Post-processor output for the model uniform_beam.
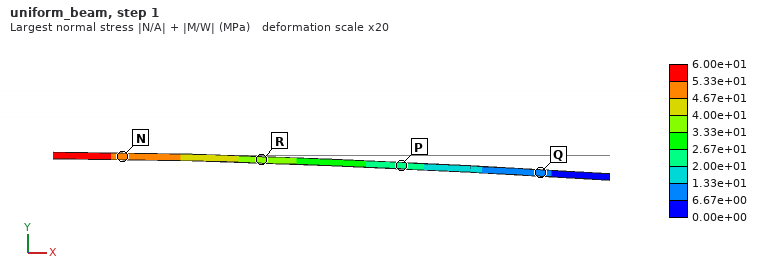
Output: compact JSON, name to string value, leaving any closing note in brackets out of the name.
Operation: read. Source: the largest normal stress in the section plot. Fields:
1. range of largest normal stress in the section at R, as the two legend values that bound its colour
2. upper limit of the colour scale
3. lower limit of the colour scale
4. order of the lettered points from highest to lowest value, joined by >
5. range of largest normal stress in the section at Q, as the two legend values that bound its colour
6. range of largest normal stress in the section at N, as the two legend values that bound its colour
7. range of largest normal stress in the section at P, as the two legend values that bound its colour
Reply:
{"range of largest normal stress in the section at R, as the two legend values that bound its colour": "3.33e+01 to 4.00e+01 MPa", "upper limit of the colour scale": "6.00e+01 MPa", "lower limit of the colour scale": "0.00e+00 MPa", "order of the lettered points from highest to lowest value, joined by >": "N > R > P > Q", "range of largest normal stress in the section at Q, as the two legend values that bound its colour": "6.67e+00 to 1.33e+01 MPa", "range of largest normal stress in the section at N, as the two legend values that bound its colour": "4.67e+01 to 5.33e+01 MPa", "range of largest normal stress in the section at P, as the two legend values that bound its colour": "2.00e+01 to 2.67e+01 MPa"}
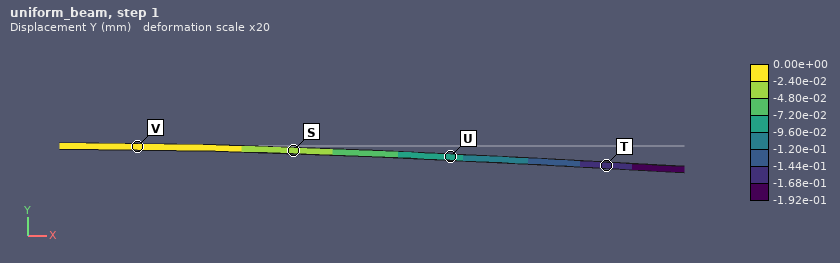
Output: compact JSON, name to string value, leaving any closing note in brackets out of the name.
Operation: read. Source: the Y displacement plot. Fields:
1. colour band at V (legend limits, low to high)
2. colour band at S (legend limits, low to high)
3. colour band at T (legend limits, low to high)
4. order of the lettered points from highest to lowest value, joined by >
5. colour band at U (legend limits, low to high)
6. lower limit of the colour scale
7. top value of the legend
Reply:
{"colour band at V": "-2.40e-02 to 0.00e+00 mm", "colour band at S": "-4.80e-02 to -2.40e-02 mm", "colour band at T": "-1.68e-01 to -1.44e-01 mm", "order of the lettered points from highest to lowest value, joined by >": "V > S > U > T", "colour band at U": "-9.60e-02 to -7.20e-02 mm", "lower limit of the colour scale": "-1.92e-01 mm", "top value of the legend": "0.00e+00 mm"}
